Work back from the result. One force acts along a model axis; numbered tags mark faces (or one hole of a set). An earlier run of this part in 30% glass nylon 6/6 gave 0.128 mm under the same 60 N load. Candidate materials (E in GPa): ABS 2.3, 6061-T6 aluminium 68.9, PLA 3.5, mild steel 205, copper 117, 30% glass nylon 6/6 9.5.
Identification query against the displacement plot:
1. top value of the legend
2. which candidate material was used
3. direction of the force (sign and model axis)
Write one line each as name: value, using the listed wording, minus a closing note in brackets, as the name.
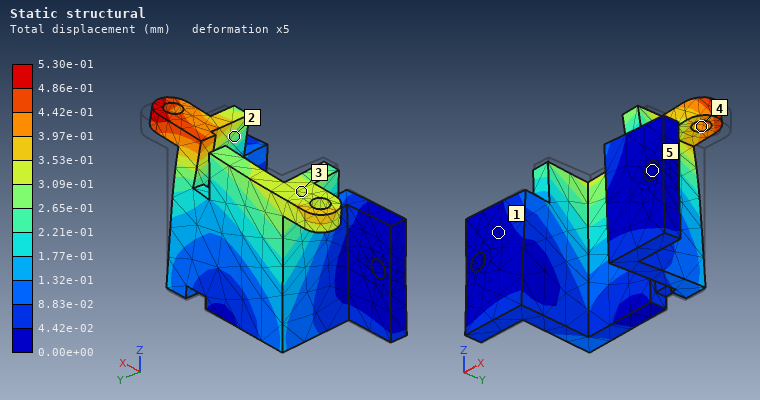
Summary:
top value of the legend: 5.30e-01 mm
which candidate material was used: ABS
direction of the force: -X
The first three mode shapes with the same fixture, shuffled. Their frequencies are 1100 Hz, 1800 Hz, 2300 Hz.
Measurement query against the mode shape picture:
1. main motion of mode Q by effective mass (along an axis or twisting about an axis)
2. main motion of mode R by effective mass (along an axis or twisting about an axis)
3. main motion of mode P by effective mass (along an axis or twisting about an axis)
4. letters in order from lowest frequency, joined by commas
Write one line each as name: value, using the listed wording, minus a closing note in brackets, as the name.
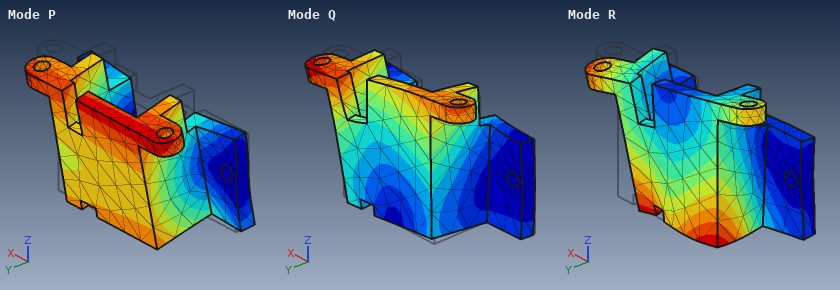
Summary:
main motion of mode Q by effective mass: along X
main motion of mode R by effective mass: along X
main motion of mode P by effective mass: along Z
letters in order from lowest frequency, joined by commas: P, Q, R
